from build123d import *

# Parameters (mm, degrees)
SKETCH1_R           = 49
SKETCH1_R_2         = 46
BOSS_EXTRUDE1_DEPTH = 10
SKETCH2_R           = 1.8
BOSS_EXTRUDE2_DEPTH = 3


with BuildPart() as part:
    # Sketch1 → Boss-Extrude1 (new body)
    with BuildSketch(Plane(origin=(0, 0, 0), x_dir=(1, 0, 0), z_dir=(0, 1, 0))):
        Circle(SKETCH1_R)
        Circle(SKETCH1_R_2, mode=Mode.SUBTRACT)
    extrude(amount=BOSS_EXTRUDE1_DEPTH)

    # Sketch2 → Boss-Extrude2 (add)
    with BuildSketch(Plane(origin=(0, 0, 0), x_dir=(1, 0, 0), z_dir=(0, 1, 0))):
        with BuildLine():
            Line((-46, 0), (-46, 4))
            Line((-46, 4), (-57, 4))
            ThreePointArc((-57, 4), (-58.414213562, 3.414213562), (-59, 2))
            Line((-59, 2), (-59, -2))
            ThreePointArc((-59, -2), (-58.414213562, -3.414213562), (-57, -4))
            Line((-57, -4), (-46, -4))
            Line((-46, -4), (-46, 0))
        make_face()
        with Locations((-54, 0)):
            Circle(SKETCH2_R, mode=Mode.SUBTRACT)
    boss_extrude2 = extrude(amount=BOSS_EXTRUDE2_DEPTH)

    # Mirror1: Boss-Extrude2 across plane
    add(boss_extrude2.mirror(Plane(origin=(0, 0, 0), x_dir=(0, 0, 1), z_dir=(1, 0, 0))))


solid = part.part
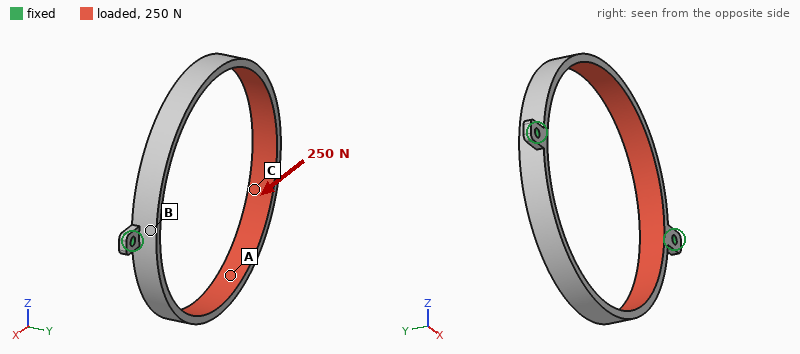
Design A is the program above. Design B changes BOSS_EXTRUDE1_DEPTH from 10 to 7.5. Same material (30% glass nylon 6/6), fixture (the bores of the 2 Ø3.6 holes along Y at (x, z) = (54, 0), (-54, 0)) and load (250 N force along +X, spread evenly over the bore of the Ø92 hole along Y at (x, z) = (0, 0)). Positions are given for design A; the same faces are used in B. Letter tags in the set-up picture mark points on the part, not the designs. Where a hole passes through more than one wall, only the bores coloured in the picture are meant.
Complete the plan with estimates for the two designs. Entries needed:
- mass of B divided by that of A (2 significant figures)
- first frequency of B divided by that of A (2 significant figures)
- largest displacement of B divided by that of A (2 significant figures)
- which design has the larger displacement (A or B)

0.76
1.0
1.3
B
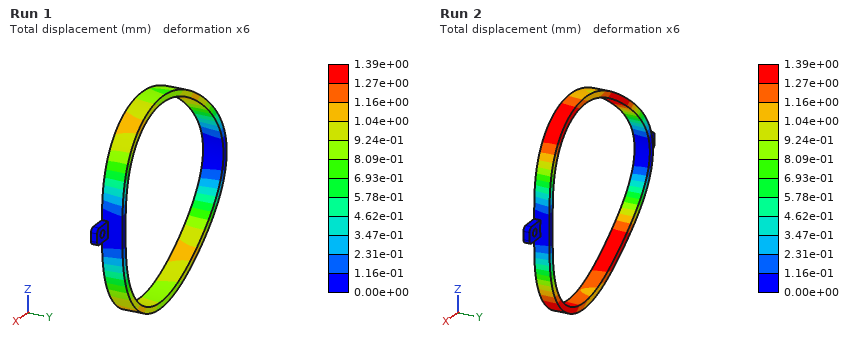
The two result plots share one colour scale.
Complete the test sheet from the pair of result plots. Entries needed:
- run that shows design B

Run 2
